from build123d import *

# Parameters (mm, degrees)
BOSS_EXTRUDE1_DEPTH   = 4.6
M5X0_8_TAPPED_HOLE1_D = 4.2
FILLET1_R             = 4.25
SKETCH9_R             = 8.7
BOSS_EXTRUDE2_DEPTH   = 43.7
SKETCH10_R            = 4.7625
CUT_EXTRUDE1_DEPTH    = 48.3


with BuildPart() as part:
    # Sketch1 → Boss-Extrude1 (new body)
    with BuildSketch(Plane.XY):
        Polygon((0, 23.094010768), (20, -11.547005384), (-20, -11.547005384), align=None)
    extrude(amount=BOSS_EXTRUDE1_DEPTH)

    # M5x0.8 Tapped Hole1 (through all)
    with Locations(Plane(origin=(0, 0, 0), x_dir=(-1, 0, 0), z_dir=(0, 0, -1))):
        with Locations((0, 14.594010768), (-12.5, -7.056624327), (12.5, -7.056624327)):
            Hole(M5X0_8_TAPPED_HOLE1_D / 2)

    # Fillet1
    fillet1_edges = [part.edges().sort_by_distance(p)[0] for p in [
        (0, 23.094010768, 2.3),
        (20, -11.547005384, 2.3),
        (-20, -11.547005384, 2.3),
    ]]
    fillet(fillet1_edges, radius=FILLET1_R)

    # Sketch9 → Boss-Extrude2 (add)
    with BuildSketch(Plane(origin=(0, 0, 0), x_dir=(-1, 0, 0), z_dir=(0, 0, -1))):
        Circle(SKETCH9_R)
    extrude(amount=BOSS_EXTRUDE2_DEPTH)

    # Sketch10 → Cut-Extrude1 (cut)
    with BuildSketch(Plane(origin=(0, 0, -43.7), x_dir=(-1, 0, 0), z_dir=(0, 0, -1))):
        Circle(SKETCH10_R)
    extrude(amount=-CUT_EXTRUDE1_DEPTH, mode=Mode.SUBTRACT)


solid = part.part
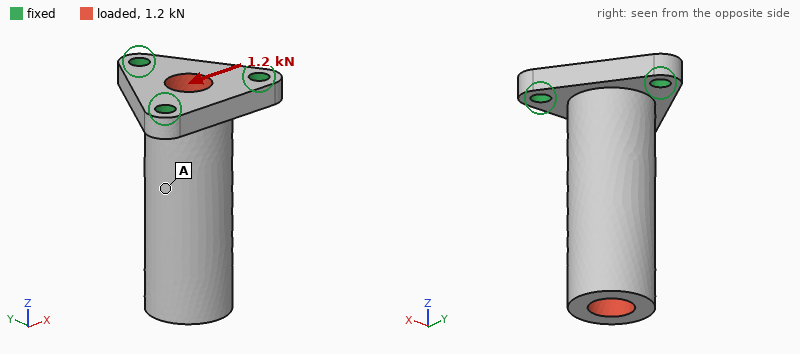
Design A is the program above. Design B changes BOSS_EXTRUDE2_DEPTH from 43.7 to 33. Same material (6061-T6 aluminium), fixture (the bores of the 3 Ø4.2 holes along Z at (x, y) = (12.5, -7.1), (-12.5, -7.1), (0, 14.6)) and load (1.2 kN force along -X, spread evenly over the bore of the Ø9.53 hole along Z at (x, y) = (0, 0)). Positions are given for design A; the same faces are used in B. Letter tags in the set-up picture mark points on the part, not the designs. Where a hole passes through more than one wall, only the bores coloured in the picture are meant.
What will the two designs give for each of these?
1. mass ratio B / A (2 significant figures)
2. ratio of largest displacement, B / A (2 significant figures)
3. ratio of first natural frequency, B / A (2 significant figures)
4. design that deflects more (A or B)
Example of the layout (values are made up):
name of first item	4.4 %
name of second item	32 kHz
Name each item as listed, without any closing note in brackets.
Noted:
mass ratio B / A	0.82
ratio of largest displacement, B / A	0.54
ratio of first natural frequency, B / A	1.5
design that deflects more	A
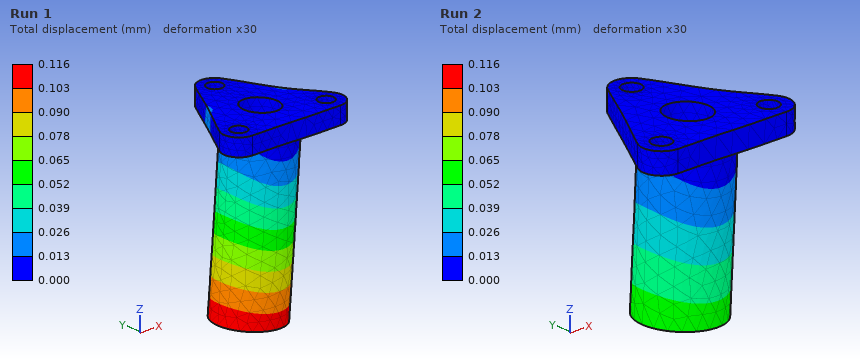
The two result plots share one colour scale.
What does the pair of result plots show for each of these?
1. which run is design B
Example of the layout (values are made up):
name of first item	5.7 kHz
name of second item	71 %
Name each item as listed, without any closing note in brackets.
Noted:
which run is design B	Run 2
